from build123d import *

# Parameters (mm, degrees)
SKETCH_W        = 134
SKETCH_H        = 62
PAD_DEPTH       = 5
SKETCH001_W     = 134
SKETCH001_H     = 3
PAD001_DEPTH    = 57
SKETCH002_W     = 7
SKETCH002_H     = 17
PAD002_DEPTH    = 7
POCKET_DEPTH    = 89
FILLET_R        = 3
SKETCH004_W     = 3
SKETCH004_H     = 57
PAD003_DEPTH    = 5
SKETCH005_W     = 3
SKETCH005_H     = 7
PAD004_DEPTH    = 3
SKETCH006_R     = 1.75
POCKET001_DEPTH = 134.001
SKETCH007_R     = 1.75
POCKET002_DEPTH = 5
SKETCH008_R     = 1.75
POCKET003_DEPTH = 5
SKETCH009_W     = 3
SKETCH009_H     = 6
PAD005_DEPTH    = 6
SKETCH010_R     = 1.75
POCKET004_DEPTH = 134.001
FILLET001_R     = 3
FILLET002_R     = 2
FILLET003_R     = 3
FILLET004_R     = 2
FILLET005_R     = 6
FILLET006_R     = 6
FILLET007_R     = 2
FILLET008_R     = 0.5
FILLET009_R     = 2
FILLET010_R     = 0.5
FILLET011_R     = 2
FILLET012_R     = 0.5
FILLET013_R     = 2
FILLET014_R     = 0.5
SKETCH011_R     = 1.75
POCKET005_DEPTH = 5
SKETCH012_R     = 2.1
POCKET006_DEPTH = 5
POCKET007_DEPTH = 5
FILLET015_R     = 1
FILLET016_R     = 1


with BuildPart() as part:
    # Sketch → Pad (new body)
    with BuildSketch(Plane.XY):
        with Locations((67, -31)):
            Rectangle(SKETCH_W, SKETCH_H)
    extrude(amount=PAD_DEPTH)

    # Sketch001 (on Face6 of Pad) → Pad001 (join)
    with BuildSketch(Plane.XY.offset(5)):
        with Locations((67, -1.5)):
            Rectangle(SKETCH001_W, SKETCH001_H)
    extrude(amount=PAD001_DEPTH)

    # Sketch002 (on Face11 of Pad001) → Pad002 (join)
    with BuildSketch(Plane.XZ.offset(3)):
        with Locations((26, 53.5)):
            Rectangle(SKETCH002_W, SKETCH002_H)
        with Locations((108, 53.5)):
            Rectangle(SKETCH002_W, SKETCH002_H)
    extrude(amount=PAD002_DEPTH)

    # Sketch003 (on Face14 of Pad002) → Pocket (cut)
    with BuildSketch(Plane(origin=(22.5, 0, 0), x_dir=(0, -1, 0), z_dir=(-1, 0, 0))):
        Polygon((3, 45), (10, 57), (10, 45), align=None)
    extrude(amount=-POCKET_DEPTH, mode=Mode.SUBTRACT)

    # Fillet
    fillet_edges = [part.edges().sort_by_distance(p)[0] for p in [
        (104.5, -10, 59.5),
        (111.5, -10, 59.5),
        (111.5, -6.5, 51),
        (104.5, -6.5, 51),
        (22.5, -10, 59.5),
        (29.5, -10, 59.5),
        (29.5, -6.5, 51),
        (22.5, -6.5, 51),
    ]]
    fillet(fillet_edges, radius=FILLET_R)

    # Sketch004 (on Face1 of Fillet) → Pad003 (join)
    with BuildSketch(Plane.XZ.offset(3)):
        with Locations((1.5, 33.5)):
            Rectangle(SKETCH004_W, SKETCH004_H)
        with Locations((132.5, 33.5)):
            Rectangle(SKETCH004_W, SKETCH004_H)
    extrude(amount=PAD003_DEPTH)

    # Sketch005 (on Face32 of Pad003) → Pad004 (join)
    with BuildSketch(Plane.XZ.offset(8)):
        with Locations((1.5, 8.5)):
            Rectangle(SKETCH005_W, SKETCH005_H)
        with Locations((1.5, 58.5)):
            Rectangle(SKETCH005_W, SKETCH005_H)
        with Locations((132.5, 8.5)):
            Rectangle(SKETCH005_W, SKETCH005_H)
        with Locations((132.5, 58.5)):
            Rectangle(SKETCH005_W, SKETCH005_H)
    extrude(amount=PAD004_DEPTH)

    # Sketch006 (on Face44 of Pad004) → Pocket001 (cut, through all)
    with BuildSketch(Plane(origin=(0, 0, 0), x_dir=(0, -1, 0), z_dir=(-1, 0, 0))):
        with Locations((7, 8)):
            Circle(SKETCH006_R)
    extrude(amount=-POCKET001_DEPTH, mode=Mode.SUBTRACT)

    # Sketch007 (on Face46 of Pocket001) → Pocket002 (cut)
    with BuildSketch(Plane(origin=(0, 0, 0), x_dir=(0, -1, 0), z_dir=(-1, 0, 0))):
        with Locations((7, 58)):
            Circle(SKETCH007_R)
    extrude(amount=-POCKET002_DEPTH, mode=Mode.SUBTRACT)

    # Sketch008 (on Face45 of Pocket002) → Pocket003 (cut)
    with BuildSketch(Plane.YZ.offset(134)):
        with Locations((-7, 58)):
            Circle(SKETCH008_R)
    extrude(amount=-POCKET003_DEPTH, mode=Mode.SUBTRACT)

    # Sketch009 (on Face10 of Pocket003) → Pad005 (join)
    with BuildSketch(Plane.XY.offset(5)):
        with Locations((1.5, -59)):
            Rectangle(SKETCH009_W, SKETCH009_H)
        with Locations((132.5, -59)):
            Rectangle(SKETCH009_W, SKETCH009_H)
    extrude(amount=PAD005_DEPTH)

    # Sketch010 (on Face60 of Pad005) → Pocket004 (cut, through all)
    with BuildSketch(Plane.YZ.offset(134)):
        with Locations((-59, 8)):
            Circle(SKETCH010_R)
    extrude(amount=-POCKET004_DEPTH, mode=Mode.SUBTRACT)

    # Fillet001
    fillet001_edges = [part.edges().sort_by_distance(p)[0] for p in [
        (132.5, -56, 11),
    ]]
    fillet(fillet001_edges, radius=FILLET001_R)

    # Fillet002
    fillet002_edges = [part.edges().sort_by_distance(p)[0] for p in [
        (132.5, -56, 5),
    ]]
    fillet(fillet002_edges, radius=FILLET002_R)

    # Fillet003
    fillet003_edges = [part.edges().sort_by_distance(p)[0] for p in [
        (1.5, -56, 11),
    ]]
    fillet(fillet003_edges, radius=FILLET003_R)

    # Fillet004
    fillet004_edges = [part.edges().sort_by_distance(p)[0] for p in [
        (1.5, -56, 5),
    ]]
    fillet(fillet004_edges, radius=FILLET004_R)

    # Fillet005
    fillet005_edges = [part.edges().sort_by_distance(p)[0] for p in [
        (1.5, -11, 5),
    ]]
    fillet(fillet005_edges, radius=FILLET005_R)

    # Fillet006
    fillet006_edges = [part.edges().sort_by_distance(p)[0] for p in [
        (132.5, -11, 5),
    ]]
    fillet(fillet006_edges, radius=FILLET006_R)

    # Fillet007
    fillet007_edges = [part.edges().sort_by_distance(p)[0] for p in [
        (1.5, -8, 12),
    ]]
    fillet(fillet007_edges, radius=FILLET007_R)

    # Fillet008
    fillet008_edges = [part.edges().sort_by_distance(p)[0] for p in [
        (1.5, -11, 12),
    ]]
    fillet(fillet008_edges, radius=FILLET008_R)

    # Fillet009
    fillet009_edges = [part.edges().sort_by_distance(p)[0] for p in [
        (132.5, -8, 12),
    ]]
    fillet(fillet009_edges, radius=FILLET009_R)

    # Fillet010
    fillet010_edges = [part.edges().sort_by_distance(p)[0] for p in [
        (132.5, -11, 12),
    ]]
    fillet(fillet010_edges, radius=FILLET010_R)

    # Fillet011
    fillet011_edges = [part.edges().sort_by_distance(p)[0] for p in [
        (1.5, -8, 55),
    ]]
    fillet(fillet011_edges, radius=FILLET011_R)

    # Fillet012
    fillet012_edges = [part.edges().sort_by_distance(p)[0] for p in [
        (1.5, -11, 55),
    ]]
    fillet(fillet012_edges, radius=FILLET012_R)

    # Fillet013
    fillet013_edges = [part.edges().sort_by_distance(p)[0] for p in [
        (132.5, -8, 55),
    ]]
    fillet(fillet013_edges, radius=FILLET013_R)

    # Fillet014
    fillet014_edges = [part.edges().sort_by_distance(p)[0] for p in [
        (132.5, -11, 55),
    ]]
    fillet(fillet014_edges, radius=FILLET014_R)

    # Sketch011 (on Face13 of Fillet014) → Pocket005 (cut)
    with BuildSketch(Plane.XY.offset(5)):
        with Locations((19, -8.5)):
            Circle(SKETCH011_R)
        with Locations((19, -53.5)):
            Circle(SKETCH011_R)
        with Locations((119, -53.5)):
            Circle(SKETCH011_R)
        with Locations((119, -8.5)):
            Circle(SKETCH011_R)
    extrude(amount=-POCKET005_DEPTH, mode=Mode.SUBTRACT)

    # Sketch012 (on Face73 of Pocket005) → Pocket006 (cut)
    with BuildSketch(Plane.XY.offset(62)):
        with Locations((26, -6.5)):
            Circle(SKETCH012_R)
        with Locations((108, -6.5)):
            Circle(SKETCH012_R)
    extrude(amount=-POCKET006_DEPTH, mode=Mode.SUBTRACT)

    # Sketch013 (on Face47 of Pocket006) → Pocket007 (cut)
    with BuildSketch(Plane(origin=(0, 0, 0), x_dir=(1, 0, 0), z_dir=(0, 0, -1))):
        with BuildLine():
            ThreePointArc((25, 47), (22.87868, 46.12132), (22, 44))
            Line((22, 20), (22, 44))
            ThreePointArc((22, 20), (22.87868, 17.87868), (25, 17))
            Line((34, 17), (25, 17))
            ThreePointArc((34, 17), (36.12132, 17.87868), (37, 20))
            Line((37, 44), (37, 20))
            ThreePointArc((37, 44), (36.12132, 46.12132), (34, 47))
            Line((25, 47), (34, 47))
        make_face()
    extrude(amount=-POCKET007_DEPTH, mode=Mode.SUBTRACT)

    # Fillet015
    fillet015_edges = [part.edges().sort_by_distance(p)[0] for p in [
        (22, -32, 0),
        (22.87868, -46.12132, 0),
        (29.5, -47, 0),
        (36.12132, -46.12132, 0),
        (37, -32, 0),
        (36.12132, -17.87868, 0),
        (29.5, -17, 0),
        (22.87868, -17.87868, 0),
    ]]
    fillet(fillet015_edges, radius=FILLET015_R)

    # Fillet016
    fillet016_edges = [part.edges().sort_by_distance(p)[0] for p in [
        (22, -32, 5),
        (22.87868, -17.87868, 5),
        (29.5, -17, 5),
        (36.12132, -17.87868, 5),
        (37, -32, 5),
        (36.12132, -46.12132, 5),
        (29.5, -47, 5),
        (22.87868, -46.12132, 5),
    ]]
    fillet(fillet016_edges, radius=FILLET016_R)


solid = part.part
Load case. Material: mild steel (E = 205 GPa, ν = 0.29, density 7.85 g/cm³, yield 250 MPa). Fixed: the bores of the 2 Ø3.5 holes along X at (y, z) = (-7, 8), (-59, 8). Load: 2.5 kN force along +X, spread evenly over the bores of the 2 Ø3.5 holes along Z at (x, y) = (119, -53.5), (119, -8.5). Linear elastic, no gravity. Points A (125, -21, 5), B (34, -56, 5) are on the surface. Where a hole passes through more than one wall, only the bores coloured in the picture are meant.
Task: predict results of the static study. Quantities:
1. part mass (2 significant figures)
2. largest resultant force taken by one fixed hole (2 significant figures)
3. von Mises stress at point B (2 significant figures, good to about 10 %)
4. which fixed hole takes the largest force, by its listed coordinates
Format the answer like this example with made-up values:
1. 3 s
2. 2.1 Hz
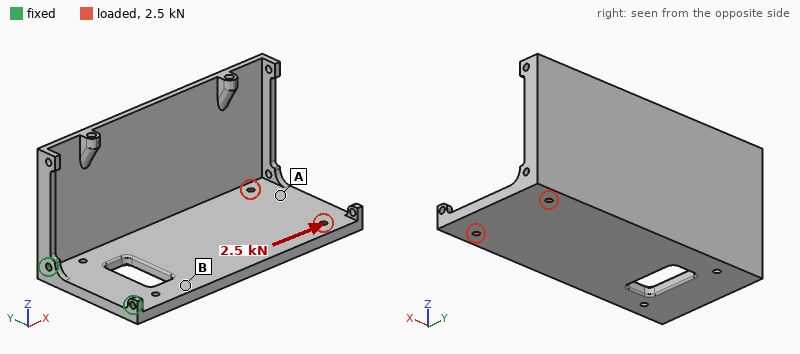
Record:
1. 510 g
2. 1.4 kN
3. 20 MPa
4. (-7, 8)
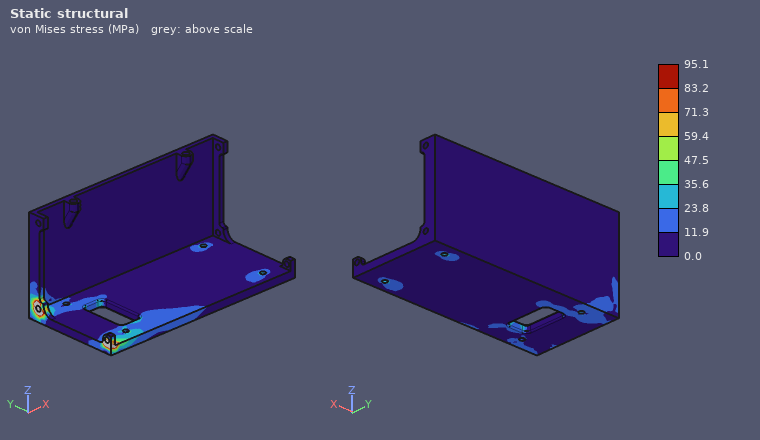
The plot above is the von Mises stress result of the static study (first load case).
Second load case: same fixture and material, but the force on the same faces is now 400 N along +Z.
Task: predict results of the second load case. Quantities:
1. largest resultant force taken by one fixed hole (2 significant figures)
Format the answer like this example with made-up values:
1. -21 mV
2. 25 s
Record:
1. 280 N
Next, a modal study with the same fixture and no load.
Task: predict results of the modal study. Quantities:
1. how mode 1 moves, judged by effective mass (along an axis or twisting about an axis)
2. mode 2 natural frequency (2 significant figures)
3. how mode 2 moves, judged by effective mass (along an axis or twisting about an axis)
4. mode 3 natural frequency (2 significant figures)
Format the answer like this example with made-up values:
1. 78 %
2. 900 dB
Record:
1. along Z
2. 440 Hz
3. along Y
4. 1100 Hz
